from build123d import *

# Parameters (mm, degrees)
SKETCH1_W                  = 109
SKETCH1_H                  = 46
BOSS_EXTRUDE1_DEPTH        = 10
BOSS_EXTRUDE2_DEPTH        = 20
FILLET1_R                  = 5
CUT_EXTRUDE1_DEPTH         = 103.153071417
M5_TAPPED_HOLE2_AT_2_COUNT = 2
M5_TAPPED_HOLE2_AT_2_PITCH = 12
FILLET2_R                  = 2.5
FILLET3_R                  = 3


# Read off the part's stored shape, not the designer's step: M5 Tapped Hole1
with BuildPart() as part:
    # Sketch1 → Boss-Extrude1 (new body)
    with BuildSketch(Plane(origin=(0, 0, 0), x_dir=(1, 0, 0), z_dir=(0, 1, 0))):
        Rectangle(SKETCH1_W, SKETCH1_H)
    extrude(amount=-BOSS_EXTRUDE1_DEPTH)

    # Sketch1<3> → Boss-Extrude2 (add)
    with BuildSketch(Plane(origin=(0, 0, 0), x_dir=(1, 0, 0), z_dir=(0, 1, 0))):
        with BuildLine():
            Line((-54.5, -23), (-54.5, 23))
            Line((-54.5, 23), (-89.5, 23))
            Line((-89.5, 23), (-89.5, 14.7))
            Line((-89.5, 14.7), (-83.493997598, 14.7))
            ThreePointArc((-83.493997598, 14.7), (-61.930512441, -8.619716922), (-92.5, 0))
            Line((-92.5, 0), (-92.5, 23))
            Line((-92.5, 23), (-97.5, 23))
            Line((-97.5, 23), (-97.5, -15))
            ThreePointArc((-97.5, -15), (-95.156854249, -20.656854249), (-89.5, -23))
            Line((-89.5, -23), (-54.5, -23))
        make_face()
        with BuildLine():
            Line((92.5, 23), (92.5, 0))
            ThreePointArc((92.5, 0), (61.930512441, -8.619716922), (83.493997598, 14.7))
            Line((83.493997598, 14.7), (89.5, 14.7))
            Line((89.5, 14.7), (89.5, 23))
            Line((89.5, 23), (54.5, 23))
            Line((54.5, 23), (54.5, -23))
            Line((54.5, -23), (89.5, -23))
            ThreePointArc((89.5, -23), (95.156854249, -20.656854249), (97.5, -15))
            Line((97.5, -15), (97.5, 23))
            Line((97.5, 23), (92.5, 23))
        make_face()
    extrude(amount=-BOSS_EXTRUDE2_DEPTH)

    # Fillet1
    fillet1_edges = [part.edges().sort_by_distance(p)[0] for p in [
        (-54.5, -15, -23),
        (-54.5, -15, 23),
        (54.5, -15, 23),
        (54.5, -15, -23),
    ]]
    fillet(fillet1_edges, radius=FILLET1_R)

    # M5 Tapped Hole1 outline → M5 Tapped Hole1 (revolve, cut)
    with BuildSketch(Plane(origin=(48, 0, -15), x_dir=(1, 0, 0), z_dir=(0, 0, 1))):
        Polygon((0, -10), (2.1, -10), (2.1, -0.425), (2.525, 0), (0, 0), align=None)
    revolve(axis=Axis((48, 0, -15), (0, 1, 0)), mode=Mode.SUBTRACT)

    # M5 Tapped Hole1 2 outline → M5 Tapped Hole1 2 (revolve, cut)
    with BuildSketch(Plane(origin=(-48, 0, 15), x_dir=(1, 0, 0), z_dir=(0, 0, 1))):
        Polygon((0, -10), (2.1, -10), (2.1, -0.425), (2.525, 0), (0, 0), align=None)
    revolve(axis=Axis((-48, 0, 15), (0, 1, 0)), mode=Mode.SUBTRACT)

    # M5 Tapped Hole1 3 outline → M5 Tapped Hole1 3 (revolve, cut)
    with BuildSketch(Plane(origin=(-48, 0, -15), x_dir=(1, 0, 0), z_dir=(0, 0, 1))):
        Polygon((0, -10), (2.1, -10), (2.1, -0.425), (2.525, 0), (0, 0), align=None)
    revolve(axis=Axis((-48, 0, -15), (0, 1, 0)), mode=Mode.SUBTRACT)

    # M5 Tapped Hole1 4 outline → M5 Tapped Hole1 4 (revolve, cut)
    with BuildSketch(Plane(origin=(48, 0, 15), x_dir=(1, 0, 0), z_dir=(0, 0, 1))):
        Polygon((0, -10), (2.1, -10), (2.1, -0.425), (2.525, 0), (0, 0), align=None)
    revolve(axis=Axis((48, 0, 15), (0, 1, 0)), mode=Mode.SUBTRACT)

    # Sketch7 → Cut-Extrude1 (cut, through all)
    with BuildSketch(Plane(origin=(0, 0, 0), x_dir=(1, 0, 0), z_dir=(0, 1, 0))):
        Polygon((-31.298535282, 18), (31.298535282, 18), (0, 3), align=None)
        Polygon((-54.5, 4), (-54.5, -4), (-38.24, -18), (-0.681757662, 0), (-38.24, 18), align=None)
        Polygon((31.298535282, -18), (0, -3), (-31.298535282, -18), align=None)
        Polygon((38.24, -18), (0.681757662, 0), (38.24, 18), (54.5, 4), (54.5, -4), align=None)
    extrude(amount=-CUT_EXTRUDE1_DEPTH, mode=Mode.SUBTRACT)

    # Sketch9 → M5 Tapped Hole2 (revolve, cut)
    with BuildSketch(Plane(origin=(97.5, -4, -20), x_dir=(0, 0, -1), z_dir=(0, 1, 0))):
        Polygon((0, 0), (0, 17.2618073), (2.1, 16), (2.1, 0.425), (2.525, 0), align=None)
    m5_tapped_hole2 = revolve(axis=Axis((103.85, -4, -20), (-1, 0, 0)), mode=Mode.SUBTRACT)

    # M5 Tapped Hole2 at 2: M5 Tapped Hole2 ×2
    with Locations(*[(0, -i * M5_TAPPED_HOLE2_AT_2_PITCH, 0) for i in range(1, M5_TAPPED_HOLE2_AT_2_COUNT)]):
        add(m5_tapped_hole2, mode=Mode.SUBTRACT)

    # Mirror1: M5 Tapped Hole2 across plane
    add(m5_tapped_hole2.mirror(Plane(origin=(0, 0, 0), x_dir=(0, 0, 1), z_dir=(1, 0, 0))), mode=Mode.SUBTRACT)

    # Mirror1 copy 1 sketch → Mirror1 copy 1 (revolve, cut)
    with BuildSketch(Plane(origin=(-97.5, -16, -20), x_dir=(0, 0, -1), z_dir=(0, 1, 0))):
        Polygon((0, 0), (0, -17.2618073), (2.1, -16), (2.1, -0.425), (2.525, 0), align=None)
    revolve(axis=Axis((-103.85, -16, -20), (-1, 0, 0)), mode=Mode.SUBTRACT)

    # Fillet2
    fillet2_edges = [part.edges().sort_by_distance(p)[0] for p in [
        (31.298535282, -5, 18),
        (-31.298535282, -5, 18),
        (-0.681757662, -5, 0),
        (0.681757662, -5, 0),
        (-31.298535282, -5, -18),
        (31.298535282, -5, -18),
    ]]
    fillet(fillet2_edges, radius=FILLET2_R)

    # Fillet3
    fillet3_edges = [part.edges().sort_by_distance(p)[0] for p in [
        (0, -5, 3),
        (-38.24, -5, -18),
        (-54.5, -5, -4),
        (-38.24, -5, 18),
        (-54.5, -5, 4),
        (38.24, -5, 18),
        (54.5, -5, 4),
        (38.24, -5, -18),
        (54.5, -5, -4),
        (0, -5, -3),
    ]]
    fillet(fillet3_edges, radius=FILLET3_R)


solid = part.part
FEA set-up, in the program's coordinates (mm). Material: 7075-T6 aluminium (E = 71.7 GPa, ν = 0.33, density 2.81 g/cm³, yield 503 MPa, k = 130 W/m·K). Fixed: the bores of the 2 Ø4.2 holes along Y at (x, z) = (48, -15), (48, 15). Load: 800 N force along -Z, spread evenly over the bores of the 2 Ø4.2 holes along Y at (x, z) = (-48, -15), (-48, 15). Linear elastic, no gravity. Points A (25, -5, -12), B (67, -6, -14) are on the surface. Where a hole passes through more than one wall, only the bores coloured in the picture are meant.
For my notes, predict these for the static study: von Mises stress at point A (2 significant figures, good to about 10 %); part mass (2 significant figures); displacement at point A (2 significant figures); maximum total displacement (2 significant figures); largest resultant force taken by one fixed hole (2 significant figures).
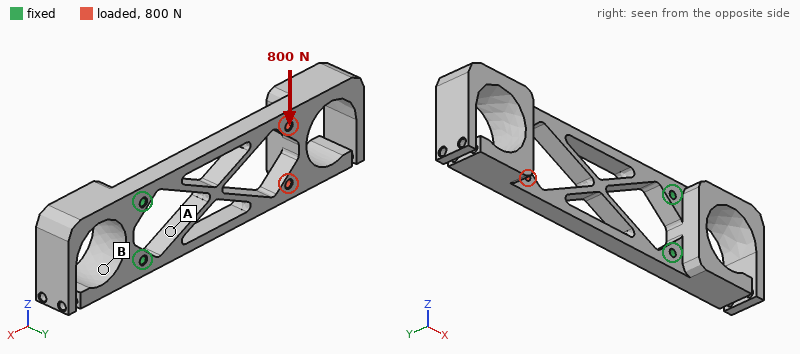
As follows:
24 MPa
170 g
0.038 mm
0.24 mm
2.0 kN
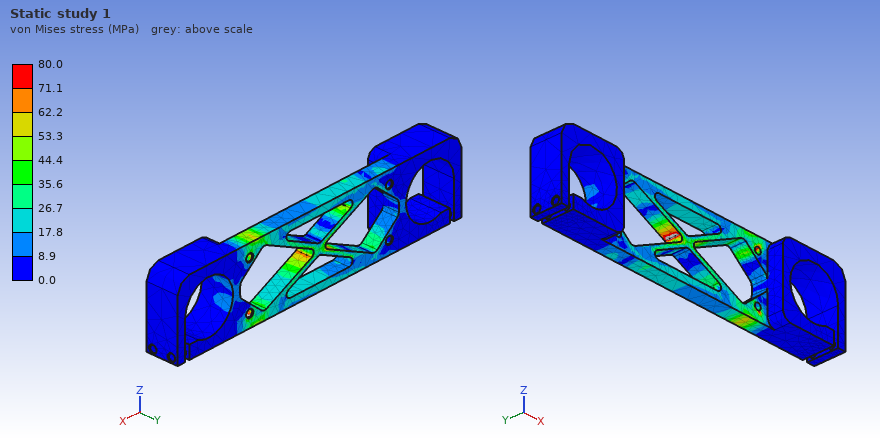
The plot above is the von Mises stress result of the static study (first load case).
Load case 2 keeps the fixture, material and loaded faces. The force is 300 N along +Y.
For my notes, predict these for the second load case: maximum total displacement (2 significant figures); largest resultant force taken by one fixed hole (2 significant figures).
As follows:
1.9 mm
150 N
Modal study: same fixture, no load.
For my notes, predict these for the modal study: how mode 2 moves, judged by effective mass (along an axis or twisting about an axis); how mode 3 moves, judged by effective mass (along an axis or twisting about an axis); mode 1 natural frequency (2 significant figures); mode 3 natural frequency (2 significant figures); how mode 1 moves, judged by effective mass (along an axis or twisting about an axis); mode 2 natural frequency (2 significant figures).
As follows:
along Z
along Z
230 Hz
1000 Hz
along Y
850 Hz
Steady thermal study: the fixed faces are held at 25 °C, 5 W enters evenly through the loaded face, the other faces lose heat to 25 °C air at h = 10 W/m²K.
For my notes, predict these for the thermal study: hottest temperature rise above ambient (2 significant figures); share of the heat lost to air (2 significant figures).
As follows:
16 K
40 %
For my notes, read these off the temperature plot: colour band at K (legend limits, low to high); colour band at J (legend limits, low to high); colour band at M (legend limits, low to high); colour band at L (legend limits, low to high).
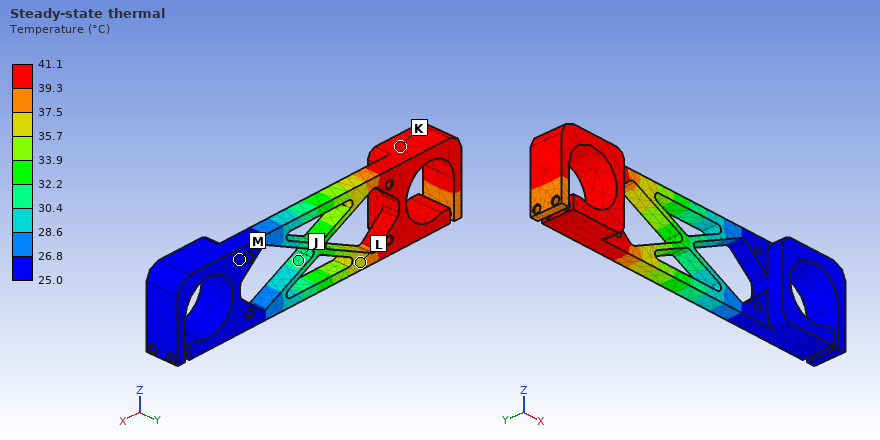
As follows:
39.3 to 41.1 °C
30.4 to 32.2 °C
25.0 to 26.8 °C
35.7 to 37.5 °C
